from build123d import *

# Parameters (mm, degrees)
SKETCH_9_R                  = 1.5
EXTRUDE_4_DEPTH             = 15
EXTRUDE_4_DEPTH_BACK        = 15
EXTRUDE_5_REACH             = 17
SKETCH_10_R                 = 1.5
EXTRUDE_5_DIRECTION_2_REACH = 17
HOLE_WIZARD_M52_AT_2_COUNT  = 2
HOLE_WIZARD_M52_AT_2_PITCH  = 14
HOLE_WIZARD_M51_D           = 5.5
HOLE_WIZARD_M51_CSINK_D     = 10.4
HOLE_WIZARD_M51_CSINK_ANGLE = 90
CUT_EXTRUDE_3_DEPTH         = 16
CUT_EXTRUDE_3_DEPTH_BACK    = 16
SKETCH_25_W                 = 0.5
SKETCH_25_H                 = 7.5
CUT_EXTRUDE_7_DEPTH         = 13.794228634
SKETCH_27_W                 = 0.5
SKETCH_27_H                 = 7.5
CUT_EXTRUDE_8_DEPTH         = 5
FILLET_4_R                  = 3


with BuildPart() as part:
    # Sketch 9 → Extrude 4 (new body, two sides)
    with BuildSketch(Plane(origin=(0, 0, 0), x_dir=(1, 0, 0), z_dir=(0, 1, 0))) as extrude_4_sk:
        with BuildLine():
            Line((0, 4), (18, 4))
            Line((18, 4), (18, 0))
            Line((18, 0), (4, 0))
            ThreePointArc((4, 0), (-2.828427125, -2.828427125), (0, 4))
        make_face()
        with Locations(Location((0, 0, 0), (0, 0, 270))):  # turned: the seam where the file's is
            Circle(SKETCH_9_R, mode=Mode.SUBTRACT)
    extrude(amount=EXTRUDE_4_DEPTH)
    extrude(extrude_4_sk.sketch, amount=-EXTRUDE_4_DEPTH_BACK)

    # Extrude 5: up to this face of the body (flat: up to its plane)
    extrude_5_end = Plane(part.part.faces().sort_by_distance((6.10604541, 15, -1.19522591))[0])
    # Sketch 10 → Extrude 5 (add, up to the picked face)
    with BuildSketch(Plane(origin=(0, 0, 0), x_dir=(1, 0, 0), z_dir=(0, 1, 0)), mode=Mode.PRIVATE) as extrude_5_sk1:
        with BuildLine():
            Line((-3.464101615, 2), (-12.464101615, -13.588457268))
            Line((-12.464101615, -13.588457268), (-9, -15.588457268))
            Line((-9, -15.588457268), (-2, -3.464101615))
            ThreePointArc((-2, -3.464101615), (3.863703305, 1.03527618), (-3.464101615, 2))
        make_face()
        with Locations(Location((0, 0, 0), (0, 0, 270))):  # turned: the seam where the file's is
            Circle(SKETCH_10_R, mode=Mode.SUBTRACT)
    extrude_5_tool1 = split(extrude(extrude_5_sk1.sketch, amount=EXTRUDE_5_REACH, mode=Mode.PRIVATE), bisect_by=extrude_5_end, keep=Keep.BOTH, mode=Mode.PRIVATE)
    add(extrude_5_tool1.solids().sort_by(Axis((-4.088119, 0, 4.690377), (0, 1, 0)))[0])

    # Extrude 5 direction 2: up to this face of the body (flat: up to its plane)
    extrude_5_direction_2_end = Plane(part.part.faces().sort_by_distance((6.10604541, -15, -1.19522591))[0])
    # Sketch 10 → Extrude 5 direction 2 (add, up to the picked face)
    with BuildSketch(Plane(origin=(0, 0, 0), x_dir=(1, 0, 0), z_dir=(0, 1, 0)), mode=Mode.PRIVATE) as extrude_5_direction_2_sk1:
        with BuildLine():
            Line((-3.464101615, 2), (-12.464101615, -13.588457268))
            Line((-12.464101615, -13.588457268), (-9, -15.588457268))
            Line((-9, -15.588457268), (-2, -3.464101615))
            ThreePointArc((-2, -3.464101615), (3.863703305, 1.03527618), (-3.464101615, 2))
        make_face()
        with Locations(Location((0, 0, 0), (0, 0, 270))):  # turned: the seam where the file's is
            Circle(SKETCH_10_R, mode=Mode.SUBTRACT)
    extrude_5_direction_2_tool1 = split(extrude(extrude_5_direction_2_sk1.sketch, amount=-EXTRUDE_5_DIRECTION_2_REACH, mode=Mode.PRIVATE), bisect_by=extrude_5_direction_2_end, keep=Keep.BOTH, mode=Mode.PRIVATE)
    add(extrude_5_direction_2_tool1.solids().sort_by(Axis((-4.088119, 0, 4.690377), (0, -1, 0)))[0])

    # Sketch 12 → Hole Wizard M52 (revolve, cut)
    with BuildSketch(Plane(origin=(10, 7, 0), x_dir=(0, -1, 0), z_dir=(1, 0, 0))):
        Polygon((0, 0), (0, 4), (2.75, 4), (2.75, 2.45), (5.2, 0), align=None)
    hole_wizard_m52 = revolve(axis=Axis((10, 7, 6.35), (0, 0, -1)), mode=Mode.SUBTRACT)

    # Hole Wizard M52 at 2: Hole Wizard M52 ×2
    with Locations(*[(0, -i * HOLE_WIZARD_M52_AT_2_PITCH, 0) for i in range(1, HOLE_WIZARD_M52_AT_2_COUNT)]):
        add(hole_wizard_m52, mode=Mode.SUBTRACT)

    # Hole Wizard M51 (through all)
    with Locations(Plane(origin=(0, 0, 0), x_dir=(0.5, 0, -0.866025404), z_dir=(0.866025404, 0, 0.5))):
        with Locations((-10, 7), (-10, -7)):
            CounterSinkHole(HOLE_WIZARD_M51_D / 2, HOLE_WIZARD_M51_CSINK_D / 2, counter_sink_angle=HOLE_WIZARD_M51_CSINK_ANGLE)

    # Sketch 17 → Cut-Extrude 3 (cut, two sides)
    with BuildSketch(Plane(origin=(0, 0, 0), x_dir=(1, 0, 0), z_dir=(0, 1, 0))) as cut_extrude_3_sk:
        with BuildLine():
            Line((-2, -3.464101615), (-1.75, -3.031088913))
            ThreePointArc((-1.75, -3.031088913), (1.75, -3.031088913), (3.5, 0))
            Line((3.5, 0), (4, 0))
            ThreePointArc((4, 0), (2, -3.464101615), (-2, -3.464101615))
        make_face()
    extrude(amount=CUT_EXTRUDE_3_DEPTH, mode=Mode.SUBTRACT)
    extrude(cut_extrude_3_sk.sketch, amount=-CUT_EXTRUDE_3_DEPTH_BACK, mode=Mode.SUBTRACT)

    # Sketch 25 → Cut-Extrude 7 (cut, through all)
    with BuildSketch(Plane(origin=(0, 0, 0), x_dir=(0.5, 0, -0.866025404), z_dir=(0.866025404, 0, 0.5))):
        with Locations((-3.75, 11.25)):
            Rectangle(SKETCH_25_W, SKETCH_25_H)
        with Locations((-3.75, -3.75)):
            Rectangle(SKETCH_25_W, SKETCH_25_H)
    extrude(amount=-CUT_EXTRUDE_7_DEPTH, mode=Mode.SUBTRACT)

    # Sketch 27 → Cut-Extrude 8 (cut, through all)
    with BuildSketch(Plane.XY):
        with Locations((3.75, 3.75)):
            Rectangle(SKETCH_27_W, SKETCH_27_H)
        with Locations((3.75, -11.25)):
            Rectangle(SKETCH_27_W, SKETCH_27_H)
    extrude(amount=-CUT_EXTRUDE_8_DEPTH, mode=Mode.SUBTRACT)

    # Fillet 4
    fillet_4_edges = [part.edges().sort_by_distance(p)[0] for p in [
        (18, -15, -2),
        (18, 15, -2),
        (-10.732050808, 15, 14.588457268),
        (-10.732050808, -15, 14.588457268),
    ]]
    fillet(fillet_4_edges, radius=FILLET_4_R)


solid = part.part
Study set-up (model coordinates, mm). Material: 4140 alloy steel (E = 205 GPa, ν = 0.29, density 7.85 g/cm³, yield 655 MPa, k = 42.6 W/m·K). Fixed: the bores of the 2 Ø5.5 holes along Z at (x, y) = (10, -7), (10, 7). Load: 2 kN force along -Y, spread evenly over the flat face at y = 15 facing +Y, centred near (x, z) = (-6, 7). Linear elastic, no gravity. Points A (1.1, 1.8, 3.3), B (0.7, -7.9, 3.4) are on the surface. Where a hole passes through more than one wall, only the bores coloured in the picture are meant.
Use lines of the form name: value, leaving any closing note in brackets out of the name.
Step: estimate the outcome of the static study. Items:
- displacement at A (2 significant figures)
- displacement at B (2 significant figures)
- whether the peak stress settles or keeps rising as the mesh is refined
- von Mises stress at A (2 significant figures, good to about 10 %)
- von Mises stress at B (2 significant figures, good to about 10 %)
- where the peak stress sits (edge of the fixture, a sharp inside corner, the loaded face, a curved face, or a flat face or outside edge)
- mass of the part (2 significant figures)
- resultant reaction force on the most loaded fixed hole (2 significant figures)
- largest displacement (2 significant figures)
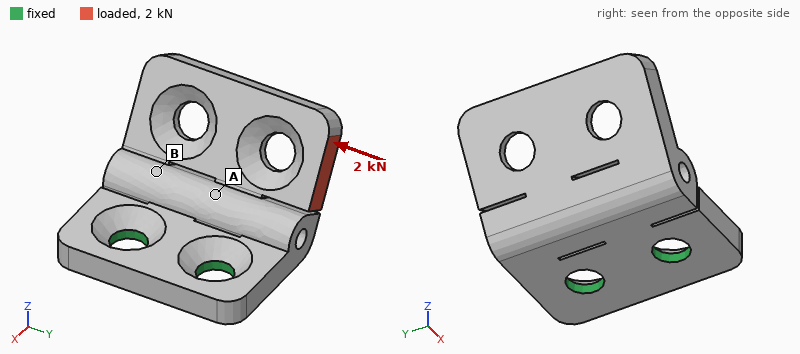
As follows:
displacement at A: 15 µm
displacement at B: 20 µm
whether the peak stress settles or keeps rising as the mesh is refined: keeps rising
von Mises stress at A: 110 MPa
von Mises stress at B: 50 MPa
where the peak stress sits: a sharp inside corner
mass of the part: 31 g
resultant reaction force on the most loaded fixed hole: 2.6 kN
largest displacement: 72 µm
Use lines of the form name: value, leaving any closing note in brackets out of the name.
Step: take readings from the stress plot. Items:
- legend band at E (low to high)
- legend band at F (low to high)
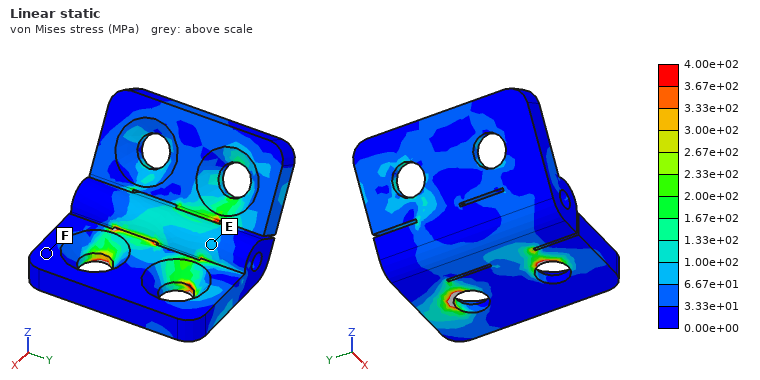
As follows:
legend band at E: 6.67e+01 to 1.00e+02 MPa
legend band at F: 0.00e+00 to 3.33e+01 MPa
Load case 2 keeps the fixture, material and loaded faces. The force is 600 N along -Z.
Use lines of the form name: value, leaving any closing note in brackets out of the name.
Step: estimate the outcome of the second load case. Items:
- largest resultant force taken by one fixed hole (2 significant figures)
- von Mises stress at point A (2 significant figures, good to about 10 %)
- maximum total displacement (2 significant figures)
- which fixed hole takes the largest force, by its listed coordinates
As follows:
largest resultant force taken by one fixed hole: 880 N
von Mises stress at point A: 81 MPa
maximum total displacement: 0.17 mm
which fixed hole takes the largest force, by its listed coordinates: (10, 7)
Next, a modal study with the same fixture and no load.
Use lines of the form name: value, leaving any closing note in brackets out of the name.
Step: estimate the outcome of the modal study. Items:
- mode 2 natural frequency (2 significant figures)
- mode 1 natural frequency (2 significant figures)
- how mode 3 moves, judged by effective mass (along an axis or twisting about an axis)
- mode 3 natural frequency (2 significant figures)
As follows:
mode 2 natural frequency: 7100 Hz
mode 1 natural frequency: 3100 Hz
how mode 3 moves, judged by effective mass: along Y
mode 3 natural frequency: 10 kHz
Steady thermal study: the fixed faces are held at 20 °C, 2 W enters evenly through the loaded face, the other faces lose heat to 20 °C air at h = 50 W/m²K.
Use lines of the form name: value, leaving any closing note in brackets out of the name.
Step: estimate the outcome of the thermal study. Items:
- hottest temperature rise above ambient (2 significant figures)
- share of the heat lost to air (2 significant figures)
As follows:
hottest temperature rise above ambient: 22 K
share of the heat lost to air: 40 %
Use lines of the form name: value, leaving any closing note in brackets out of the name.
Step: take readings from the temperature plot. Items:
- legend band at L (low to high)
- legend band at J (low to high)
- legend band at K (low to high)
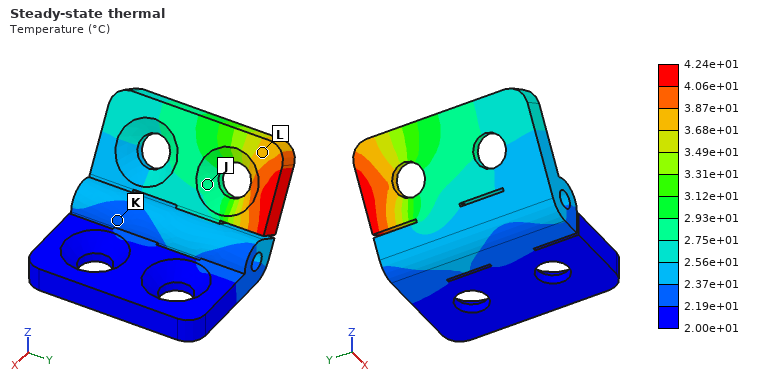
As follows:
legend band at L: 3.68e+01 to 3.87e+01 °C
legend band at J: 2.75e+01 to 2.93e+01 °C
legend band at K: 2.19e+01 to 2.37e+01 °C
